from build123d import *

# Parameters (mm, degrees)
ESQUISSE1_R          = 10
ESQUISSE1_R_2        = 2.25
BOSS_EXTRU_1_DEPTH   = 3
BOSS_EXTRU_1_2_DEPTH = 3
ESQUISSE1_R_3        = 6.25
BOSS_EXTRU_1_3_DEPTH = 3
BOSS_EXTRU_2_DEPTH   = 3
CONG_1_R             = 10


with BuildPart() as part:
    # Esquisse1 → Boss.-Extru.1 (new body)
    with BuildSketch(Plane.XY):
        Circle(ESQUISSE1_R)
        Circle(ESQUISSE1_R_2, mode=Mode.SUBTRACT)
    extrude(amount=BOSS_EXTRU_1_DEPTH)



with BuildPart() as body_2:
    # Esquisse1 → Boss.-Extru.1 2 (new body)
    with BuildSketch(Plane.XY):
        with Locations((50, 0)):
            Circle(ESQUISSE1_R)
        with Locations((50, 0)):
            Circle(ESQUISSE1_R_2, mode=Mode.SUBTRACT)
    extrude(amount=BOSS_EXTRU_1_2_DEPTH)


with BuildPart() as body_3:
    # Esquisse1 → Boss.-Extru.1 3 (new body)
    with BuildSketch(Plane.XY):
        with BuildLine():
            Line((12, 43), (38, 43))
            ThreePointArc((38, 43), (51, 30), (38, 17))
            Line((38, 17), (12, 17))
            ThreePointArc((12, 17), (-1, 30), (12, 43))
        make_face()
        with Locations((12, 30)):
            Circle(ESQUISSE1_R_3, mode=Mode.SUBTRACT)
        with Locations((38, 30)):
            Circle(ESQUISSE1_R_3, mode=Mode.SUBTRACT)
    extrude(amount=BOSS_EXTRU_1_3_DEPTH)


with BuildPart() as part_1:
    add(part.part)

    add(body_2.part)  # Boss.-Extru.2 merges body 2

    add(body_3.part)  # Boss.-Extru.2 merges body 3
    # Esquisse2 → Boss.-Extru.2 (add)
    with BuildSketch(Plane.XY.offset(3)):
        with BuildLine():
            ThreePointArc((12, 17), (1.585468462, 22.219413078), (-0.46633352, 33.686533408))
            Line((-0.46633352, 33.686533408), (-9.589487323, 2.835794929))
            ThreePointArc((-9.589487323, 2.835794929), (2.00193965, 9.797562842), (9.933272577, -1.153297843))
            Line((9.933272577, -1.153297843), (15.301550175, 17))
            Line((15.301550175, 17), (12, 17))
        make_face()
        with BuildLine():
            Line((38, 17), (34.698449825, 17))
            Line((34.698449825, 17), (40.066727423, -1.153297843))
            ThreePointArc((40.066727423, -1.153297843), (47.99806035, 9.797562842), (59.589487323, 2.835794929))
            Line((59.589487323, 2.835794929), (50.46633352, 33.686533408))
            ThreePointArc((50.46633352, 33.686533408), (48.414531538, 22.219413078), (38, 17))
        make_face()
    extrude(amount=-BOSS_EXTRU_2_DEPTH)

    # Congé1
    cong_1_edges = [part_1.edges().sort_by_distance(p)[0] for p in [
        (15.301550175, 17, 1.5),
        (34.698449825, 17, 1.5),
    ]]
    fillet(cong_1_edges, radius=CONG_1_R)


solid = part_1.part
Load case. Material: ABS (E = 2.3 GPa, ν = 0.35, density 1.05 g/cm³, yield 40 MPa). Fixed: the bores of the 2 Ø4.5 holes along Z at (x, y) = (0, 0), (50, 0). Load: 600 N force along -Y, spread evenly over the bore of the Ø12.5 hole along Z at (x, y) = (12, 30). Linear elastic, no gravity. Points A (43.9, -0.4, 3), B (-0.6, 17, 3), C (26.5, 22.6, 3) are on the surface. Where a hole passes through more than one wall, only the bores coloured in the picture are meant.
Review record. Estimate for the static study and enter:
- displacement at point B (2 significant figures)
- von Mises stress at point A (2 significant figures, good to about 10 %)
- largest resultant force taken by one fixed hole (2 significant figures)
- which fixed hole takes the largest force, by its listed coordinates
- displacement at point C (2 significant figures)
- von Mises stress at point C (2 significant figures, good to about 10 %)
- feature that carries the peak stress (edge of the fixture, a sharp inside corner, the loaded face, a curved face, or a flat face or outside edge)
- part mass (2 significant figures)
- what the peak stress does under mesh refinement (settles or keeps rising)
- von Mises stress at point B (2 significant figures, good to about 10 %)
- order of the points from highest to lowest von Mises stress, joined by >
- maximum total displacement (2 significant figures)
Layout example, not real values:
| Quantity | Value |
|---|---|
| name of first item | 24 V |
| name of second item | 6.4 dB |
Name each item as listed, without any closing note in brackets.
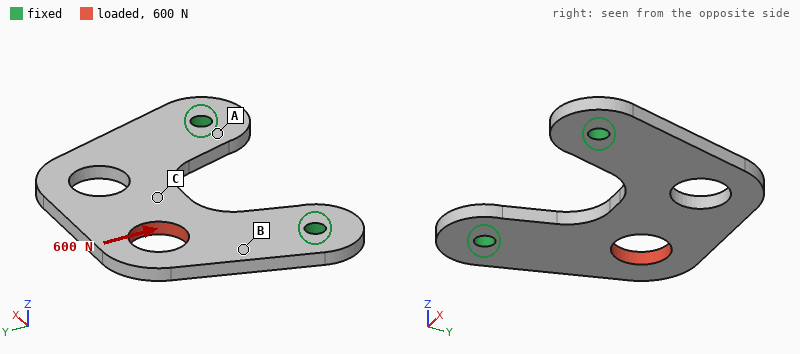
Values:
| Quantity | Value |
|---|---|
| displacement at point B | 0.066 mm |
| von Mises stress at point A | 2.2 MPa |
| largest resultant force taken by one fixed hole | 480 N |
| which fixed hole takes the largest force, by its listed coordinates | (0, 0) |
| displacement at point C | 0.11 mm |
| von Mises stress at point C | 5.4 MPa |
| feature that carries the peak stress | edge of the fixture |
| part mass | 6.6 g |
| what the peak stress does under mesh refinement | keeps rising |
| von Mises stress at point B | 8.4 MPa |
| order of the points from highest to lowest von Mises stress, joined by > | B > C > A |
| maximum total displacement | 0.19 mm |
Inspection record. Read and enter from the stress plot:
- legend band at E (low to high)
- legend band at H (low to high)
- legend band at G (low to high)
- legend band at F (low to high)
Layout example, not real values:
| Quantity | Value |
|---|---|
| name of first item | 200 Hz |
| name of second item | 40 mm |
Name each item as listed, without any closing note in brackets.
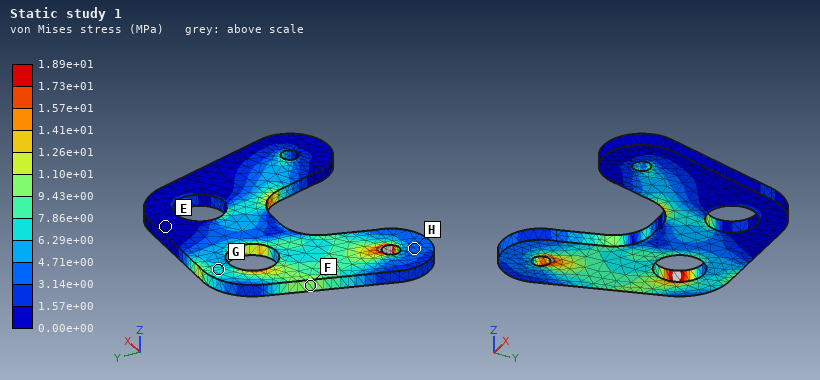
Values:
| Quantity | Value |
|---|---|
| legend band at E | 0.00e+00 to 1.57e+00 MPa |
| legend band at H | 3.14e+00 to 4.71e+00 MPa |
| legend band at G | 6.29e+00 to 7.86e+00 MPa |
| legend band at F | 9.43e+00 to 1.10e+01 MPa |
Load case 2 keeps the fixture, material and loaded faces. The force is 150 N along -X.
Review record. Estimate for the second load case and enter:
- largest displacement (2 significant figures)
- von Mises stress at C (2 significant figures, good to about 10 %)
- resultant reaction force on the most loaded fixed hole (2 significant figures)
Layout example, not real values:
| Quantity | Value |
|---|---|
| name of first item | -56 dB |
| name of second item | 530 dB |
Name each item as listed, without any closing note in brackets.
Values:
| Quantity | Value |
|---|---|
| largest displacement | 0.12 mm |
| von Mises stress at C | 2.2 MPa |
| resultant reaction force on the most loaded fixed hole | 110 N |
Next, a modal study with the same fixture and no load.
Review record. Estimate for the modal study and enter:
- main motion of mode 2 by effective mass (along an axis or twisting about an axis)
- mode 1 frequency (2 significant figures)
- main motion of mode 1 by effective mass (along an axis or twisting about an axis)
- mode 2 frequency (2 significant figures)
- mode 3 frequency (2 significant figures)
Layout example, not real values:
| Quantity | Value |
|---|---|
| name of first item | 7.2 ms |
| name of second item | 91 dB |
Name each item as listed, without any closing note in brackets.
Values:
| Quantity | Value |
|---|---|
| main motion of mode 2 by effective mass | twisting about Y |
| mode 1 frequency | 380 Hz |
| main motion of mode 1 by effective mass | along Z |
| mode 2 frequency | 970 Hz |
| mode 3 frequency | 1900 Hz |
